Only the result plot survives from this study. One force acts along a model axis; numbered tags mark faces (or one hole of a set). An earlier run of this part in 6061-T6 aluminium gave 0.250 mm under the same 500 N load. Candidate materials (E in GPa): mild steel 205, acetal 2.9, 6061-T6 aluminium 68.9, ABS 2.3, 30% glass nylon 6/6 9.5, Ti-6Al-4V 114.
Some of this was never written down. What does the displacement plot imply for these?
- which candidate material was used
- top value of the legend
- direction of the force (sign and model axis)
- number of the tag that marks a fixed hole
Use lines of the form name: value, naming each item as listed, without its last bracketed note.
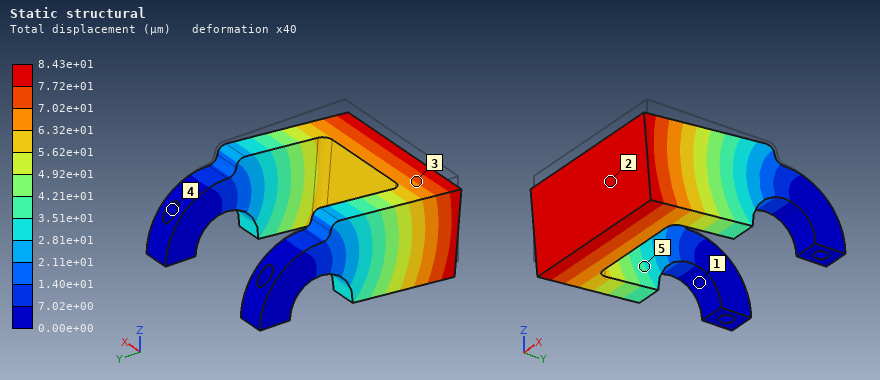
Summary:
which candidate material was used: mild steel
top value of the legend: 8.43e+01 µm
direction of the force: -Z
number of the tag that marks a fixed hole: 4
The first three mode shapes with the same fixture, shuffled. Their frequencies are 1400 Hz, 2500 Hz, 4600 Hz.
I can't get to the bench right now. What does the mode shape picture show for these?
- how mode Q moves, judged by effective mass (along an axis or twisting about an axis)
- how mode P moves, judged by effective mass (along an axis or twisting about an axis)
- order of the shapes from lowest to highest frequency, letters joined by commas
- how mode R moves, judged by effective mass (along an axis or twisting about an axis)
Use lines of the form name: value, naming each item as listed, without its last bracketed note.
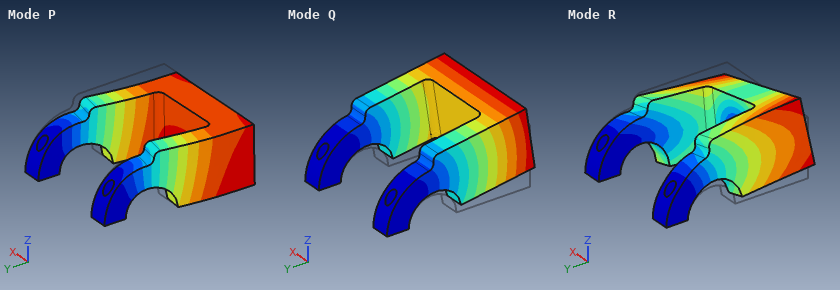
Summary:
how mode Q moves, judged by effective mass: along Z
how mode P moves, judged by effective mass: along X
order of the shapes from lowest to highest frequency, letters joined by commas: Q, P, R
how mode R moves, judged by effective mass: twisting about Y
